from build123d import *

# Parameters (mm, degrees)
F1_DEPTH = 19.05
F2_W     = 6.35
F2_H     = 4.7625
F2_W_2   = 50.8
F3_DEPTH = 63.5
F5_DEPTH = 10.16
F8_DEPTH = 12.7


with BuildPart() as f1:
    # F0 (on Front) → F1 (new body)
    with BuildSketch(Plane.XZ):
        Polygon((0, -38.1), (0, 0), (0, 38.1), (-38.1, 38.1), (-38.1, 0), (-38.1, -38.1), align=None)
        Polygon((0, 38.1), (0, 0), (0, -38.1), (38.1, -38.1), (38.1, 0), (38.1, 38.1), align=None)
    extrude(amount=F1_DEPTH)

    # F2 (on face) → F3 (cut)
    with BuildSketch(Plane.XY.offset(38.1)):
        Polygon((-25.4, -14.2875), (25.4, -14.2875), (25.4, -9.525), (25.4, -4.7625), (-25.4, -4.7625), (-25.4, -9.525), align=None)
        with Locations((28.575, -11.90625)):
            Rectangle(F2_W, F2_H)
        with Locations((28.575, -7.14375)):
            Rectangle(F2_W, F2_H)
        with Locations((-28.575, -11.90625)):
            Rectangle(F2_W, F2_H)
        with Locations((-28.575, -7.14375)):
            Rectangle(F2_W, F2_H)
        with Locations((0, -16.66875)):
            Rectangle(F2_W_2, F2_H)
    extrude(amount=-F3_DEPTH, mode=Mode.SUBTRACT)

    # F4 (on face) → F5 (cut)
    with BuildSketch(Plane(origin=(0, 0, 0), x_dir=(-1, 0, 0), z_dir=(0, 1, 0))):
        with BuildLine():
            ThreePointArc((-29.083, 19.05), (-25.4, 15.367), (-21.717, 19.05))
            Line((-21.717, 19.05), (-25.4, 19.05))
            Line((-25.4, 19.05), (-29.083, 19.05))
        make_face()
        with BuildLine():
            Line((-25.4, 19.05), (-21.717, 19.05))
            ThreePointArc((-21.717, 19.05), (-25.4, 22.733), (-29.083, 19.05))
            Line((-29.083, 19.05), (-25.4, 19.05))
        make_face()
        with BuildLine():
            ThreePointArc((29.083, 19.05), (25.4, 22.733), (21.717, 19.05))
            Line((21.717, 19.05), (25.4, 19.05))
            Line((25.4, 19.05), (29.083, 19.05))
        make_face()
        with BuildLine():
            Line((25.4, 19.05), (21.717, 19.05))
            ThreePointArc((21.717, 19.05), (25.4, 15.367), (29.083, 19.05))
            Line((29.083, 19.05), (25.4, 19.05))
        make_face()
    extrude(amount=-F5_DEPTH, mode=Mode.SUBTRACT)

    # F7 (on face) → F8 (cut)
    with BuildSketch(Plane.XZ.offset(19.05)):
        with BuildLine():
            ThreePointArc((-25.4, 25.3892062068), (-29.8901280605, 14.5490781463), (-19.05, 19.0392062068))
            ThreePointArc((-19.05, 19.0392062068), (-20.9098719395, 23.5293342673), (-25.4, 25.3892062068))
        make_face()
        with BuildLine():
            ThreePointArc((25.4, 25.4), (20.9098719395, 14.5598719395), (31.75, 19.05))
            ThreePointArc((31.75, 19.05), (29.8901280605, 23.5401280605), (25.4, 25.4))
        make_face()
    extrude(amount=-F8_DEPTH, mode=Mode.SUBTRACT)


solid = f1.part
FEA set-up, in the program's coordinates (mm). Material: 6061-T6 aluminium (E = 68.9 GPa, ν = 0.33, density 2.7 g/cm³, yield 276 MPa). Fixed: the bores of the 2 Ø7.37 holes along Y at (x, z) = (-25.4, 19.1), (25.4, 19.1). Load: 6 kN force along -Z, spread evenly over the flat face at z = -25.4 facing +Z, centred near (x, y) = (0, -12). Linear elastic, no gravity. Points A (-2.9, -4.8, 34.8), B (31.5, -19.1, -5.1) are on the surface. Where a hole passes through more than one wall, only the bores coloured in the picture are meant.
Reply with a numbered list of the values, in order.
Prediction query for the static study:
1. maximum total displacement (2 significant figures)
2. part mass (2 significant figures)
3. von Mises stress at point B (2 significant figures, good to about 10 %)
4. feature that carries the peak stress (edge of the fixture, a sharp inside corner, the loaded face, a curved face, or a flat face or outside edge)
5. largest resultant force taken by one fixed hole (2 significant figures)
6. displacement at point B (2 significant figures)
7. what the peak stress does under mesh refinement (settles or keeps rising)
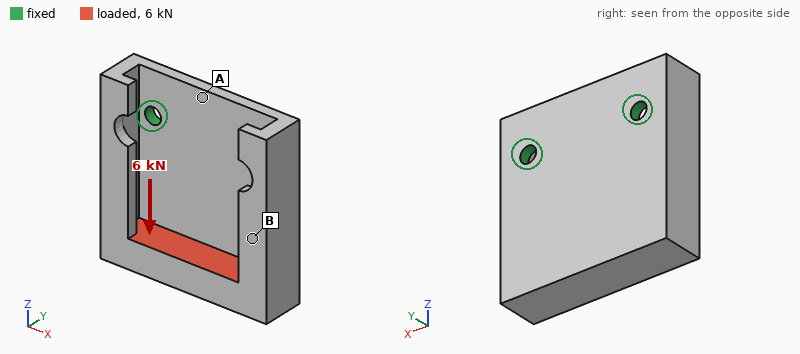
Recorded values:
1. 0.32 mm
2. 150 g
3. 31 MPa
4. edge of the fixture
5. 3.0 kN
6. 0.14 mm
7. keeps rising
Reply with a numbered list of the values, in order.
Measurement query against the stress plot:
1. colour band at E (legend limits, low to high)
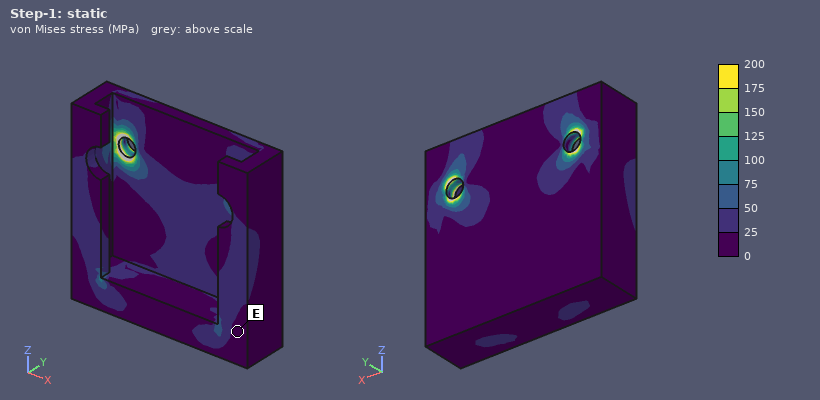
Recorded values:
1. 0 to 25 MPa
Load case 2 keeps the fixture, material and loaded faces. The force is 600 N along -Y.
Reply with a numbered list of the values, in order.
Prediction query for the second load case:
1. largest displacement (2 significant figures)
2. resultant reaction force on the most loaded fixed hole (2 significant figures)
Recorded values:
1. 0.14 mm
2. 310 N
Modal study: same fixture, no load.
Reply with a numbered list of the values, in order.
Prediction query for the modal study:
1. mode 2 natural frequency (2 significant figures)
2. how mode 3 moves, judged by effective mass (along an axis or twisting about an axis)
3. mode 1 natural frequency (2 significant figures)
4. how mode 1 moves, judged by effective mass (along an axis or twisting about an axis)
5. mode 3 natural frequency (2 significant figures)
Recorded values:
1. 2600 Hz
2. along X
3. 1300 Hz
4. along Y
5. 5800 Hz
